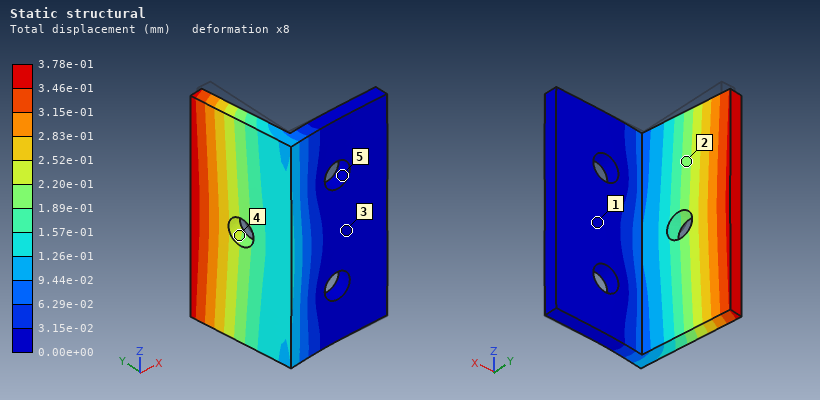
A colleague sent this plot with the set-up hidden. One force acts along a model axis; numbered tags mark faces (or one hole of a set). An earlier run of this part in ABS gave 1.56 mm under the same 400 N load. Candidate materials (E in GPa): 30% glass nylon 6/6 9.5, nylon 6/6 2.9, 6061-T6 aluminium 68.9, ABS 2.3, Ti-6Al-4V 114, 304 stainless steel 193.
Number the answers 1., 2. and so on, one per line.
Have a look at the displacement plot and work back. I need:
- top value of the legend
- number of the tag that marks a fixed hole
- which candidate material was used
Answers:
1. 3.78e-01 mm
2. 5
3. 30% glass nylon 6/6
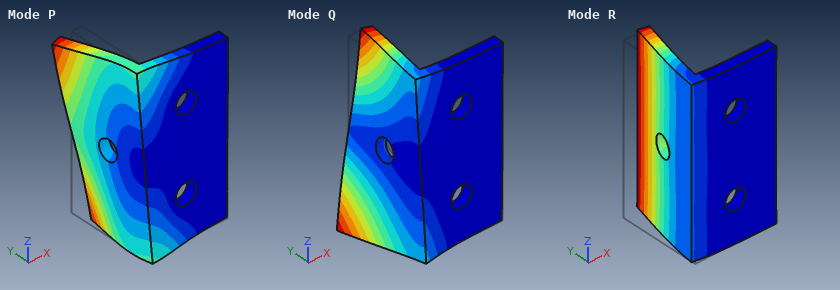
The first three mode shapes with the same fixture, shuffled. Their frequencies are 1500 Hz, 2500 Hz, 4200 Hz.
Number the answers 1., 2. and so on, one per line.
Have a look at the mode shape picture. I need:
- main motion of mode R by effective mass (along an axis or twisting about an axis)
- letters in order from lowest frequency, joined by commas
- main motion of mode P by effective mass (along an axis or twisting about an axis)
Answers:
1. along X
2. R, Q, P
3. along Z
